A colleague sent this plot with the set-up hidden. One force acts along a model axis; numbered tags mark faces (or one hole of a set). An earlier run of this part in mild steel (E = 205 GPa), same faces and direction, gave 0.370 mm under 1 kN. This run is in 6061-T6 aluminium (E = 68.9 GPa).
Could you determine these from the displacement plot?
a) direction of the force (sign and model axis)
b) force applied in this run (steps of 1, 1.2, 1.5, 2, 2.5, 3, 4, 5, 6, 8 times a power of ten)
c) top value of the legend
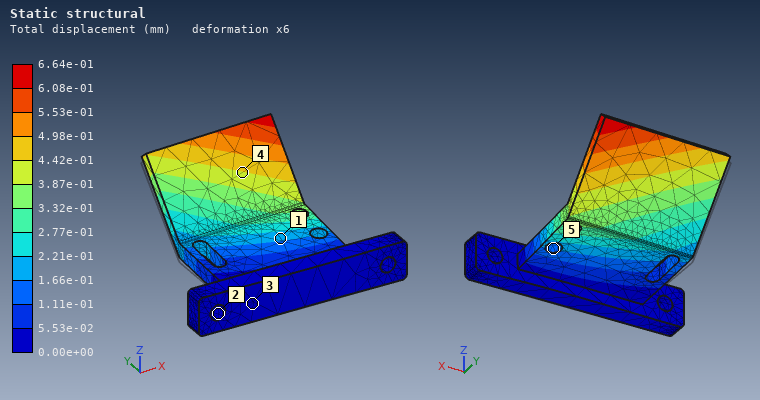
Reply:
+Z
600 N
6.64e-01 mm
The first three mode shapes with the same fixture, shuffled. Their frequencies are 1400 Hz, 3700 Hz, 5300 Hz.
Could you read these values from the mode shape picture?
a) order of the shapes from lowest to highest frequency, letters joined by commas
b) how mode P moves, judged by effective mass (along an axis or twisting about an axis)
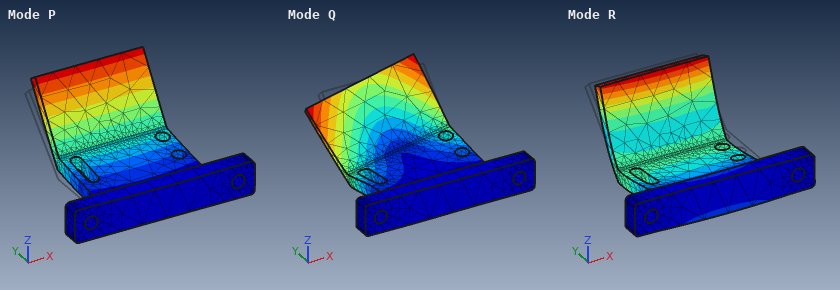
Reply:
P, Q, R
along Z
